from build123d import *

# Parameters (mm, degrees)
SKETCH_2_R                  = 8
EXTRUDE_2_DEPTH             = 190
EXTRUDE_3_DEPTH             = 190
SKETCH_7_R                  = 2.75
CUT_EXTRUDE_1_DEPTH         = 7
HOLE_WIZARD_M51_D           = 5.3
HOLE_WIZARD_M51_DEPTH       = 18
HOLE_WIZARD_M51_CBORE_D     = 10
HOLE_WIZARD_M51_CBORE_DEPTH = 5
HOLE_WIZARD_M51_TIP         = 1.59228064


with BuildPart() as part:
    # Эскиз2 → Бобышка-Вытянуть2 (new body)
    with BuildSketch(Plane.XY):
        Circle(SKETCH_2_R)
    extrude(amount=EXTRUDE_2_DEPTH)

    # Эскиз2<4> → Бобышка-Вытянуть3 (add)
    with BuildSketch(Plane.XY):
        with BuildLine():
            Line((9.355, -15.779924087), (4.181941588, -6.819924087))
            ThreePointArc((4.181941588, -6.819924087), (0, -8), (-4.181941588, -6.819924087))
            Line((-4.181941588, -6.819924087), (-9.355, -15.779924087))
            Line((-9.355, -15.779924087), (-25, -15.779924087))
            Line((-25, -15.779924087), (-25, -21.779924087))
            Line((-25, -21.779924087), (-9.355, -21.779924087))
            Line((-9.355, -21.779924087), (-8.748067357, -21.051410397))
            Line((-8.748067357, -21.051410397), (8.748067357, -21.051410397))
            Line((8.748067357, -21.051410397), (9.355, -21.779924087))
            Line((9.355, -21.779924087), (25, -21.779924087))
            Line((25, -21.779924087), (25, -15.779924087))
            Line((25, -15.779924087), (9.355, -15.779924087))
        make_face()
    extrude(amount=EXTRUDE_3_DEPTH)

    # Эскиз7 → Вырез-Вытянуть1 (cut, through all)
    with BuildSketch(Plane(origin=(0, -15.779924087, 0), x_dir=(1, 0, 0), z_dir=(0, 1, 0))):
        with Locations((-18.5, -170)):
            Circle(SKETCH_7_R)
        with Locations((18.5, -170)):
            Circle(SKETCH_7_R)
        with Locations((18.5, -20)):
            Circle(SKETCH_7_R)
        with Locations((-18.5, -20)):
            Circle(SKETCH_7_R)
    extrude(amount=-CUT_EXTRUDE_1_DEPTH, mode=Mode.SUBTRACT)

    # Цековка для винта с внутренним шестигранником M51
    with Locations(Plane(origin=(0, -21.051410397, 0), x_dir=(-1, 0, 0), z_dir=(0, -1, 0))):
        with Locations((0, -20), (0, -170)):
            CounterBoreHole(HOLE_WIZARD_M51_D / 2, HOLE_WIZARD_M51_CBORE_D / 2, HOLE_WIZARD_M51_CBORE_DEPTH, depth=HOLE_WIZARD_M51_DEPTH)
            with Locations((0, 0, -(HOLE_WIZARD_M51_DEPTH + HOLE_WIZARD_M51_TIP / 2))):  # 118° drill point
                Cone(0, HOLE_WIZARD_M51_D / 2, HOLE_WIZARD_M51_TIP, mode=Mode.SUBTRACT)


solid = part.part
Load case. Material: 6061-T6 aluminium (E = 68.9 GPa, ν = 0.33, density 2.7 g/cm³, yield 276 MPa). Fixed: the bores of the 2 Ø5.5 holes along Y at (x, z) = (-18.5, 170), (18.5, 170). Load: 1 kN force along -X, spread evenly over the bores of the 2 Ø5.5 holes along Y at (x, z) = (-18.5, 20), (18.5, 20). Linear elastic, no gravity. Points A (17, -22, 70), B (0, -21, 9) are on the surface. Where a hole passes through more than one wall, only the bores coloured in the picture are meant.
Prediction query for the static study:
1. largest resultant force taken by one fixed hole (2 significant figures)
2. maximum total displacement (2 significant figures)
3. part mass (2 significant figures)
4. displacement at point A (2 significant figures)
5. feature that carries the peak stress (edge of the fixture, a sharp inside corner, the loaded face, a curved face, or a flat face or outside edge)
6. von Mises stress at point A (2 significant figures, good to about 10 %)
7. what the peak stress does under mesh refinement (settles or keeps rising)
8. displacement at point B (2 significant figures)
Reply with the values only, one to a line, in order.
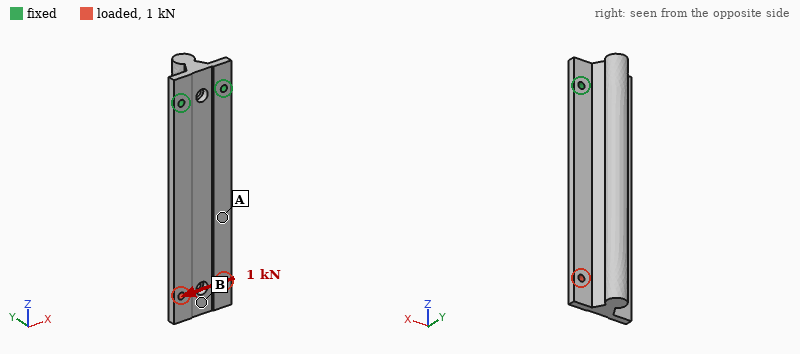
3.9 kN
0.33 mm
300 g
0.15 mm
edge of the fixture
14 MPa
keeps rising
0.30 mm
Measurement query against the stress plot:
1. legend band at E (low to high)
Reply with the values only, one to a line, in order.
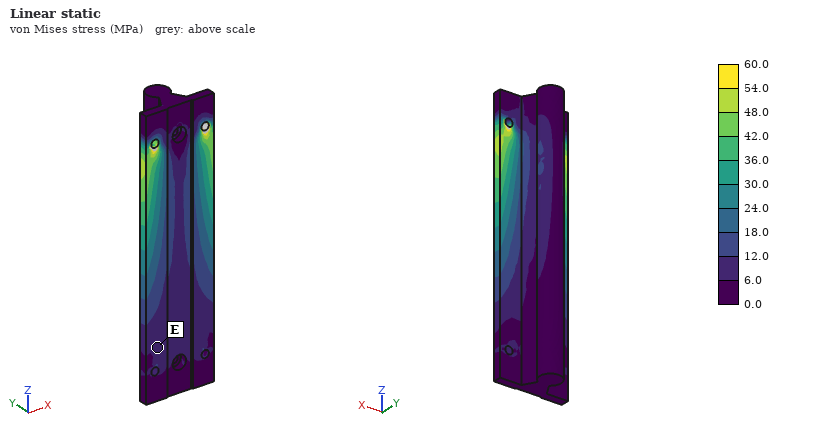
6.0 to 12.0 MPa
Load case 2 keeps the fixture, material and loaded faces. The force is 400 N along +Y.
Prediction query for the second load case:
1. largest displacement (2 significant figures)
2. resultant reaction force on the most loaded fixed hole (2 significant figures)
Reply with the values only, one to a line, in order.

1.1 mm
320 N
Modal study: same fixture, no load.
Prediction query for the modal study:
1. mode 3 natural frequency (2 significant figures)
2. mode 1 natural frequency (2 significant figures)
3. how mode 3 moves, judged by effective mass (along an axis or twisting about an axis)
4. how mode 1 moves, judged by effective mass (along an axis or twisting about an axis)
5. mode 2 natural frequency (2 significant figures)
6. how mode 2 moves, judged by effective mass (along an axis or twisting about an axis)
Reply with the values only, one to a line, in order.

1900 Hz
310 Hz
twisting about Z
along Y
970 Hz
along X
